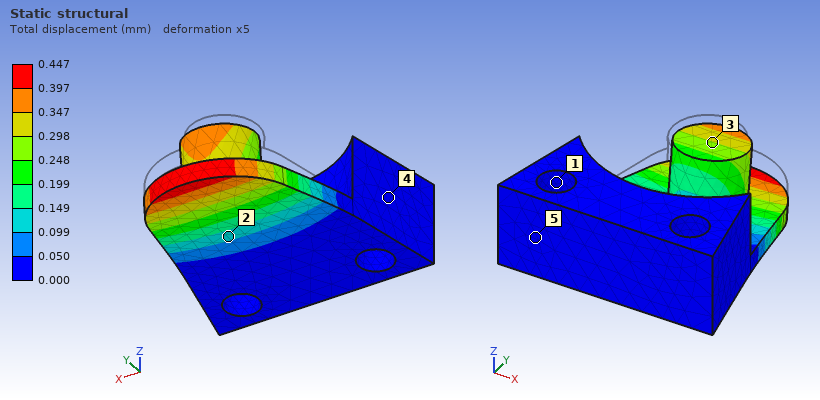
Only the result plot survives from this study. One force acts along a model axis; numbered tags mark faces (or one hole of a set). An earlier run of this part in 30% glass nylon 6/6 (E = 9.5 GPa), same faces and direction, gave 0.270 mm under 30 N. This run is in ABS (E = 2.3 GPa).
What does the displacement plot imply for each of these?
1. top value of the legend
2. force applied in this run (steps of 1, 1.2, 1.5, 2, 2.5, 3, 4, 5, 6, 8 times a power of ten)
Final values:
0.447 mm
12 N
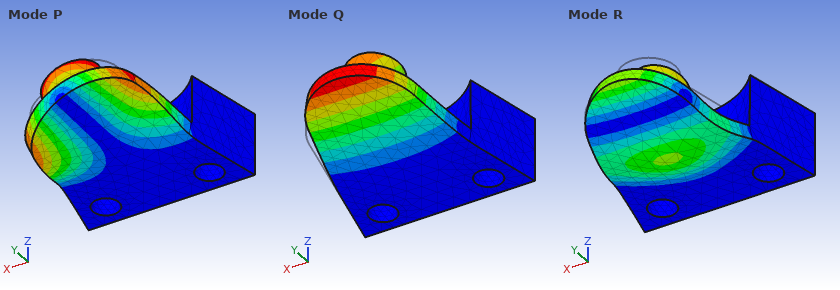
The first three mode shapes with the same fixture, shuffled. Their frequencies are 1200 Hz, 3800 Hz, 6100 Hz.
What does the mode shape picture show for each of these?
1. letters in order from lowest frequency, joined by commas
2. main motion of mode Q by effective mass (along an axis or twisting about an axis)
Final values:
Q, P, R
along Z
